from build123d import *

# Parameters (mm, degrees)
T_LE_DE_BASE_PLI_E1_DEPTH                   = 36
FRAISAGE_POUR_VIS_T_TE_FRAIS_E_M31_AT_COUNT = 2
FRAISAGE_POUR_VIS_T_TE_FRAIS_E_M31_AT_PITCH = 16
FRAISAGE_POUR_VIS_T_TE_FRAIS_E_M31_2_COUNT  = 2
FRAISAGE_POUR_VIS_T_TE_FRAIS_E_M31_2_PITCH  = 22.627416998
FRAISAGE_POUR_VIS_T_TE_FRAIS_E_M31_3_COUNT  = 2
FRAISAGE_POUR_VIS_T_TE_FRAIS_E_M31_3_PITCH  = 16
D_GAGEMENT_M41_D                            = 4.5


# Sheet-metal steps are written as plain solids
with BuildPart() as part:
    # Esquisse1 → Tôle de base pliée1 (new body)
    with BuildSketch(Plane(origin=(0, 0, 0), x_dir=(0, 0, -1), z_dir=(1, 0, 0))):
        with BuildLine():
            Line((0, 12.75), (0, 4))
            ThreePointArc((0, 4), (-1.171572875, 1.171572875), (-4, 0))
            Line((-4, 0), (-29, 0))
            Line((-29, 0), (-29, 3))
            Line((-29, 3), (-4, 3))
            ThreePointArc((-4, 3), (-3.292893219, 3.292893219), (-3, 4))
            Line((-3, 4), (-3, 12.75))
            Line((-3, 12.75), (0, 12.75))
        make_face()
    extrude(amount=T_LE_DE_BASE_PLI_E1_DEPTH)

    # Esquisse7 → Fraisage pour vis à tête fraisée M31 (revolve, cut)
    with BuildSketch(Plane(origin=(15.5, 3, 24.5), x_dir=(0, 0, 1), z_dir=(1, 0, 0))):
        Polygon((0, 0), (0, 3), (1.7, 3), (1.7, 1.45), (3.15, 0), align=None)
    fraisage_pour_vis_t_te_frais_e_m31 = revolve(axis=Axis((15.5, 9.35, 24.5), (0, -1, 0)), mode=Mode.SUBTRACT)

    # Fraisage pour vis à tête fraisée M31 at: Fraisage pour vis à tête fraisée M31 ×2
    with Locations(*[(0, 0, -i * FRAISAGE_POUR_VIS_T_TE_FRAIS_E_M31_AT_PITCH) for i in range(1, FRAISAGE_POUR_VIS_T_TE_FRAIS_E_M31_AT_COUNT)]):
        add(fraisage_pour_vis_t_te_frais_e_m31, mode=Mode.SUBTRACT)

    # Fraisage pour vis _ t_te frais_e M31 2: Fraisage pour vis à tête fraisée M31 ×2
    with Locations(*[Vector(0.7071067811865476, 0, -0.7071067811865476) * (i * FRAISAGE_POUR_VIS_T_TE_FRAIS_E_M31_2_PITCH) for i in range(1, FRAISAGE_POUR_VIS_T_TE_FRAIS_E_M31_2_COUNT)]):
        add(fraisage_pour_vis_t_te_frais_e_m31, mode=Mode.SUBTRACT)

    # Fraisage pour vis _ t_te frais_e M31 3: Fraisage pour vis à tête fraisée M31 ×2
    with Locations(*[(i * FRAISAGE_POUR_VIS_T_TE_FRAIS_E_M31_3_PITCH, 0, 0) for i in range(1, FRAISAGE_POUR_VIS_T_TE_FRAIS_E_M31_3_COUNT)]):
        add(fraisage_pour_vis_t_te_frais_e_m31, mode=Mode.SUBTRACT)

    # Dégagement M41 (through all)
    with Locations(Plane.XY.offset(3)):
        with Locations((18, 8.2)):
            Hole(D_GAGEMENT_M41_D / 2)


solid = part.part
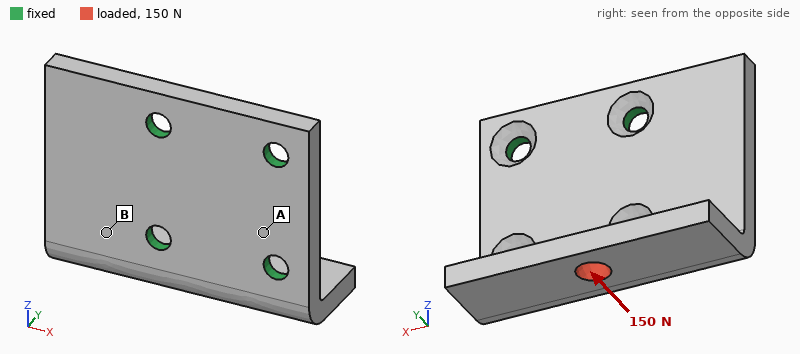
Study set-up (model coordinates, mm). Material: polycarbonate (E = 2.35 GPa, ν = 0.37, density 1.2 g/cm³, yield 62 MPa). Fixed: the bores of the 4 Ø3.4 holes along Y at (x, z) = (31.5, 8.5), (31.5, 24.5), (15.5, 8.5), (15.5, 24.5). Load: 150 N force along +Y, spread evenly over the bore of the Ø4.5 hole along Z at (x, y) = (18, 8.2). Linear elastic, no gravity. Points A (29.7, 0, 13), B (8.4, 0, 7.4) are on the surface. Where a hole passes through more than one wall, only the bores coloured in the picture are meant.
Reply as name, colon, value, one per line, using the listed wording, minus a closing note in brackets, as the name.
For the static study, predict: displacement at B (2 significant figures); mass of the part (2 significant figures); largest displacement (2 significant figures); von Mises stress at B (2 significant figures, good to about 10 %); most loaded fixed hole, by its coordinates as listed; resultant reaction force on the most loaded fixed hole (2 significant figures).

displacement at B: 0.080 mm
mass of the part: 4.6 g
largest displacement: 0.48 mm
von Mises stress at B: 9.4 MPa
most loaded fixed hole, by its coordinates as listed: (15.5, 8.5)
resultant reaction force on the most loaded fixed hole: 150 N
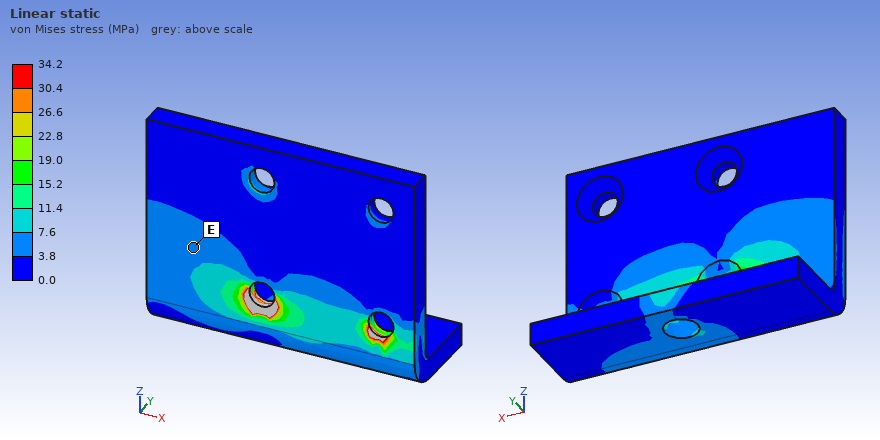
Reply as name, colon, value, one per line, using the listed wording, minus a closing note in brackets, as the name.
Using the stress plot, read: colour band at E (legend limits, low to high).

colour band at E: 3.8 to 7.6 MPa
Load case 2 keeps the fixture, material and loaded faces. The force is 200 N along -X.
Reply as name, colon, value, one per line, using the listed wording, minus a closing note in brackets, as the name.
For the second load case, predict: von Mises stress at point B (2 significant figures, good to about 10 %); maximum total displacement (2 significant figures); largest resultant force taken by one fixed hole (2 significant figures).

von Mises stress at point B: 4.2 MPa
maximum total displacement: 0.38 mm
largest resultant force taken by one fixed hole: 150 N
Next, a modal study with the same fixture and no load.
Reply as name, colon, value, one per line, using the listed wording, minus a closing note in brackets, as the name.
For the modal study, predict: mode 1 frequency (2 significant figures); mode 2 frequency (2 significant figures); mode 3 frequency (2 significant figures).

mode 1 frequency: 2200 Hz
mode 2 frequency: 2700 Hz
mode 3 frequency: 3200 Hz
